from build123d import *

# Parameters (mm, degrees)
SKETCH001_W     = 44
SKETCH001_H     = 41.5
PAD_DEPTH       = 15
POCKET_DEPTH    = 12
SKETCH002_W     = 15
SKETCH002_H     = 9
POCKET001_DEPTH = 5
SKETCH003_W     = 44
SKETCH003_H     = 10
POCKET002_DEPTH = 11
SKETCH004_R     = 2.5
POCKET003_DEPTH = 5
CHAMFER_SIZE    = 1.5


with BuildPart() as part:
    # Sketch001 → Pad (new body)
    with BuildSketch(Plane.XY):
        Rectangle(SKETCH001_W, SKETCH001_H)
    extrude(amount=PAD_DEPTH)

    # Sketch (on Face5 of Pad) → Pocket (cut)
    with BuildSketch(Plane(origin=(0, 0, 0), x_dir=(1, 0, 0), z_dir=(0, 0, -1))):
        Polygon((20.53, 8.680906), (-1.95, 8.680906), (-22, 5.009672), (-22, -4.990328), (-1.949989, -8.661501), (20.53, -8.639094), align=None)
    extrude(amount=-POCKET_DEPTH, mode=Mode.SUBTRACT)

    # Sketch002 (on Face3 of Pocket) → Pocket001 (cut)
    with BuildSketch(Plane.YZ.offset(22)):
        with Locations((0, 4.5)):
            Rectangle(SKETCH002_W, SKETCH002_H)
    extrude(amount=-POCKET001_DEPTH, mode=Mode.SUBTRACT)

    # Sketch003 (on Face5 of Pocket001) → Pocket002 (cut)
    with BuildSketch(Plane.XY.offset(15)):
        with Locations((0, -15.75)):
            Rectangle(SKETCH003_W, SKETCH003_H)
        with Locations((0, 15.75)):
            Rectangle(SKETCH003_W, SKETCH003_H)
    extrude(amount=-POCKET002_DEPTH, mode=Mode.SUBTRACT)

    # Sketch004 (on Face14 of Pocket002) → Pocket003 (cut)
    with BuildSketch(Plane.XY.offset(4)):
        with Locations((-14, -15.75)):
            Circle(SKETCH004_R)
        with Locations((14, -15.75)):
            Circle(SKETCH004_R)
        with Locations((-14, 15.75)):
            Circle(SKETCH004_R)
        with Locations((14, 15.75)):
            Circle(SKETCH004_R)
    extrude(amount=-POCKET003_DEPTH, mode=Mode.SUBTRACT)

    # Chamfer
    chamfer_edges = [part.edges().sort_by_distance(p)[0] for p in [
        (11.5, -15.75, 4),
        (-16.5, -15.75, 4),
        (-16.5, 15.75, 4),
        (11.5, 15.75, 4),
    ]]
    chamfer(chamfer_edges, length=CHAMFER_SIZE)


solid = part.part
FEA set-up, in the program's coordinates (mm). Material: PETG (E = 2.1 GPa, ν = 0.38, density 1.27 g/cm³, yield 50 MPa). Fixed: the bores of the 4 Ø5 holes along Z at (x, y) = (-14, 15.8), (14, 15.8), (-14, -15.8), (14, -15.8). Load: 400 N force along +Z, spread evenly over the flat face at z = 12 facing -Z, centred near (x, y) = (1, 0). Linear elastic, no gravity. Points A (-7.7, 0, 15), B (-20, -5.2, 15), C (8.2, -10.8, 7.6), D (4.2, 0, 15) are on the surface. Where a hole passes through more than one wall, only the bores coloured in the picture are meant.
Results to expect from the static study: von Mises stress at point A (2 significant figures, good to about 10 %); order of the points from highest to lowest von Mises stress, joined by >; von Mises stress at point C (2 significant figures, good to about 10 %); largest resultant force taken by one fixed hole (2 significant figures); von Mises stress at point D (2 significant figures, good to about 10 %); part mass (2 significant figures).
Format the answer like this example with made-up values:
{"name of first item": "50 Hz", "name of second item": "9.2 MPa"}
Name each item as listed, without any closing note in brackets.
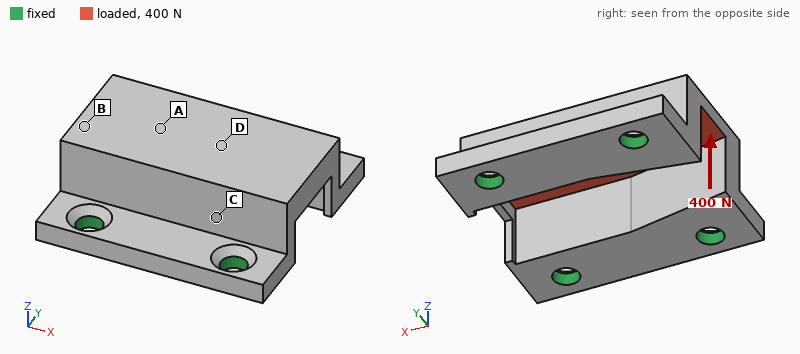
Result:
{"von Mises stress at point A": "6.5 MPa", "order of the points from highest to lowest von Mises stress, joined by >": "D > A > C > B", "von Mises stress at point C": "2.7 MPa", "largest resultant force taken by one fixed hole": "120 N", "von Mises stress at point D": "8.3 MPa", "part mass": "12 g"}
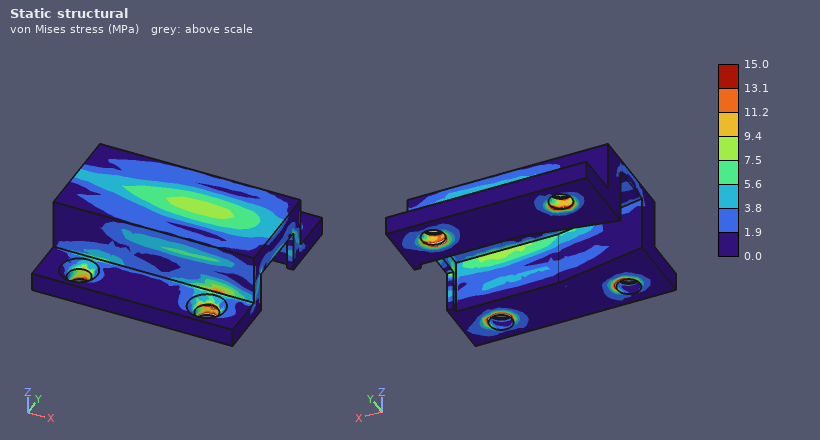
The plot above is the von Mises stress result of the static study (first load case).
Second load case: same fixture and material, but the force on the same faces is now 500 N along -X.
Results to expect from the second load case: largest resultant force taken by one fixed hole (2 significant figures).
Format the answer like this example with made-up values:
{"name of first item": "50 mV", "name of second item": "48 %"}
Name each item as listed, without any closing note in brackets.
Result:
{"largest resultant force taken by one fixed hole": "160 N"}
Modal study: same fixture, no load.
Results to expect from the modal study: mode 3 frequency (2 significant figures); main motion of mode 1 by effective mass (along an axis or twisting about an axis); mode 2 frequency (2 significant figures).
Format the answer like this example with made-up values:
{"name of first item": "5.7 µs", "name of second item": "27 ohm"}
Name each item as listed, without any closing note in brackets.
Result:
{"mode 3 frequency": "4400 Hz", "main motion of mode 1 by effective mass": "along Y", "mode 2 frequency": "4200 Hz"}
